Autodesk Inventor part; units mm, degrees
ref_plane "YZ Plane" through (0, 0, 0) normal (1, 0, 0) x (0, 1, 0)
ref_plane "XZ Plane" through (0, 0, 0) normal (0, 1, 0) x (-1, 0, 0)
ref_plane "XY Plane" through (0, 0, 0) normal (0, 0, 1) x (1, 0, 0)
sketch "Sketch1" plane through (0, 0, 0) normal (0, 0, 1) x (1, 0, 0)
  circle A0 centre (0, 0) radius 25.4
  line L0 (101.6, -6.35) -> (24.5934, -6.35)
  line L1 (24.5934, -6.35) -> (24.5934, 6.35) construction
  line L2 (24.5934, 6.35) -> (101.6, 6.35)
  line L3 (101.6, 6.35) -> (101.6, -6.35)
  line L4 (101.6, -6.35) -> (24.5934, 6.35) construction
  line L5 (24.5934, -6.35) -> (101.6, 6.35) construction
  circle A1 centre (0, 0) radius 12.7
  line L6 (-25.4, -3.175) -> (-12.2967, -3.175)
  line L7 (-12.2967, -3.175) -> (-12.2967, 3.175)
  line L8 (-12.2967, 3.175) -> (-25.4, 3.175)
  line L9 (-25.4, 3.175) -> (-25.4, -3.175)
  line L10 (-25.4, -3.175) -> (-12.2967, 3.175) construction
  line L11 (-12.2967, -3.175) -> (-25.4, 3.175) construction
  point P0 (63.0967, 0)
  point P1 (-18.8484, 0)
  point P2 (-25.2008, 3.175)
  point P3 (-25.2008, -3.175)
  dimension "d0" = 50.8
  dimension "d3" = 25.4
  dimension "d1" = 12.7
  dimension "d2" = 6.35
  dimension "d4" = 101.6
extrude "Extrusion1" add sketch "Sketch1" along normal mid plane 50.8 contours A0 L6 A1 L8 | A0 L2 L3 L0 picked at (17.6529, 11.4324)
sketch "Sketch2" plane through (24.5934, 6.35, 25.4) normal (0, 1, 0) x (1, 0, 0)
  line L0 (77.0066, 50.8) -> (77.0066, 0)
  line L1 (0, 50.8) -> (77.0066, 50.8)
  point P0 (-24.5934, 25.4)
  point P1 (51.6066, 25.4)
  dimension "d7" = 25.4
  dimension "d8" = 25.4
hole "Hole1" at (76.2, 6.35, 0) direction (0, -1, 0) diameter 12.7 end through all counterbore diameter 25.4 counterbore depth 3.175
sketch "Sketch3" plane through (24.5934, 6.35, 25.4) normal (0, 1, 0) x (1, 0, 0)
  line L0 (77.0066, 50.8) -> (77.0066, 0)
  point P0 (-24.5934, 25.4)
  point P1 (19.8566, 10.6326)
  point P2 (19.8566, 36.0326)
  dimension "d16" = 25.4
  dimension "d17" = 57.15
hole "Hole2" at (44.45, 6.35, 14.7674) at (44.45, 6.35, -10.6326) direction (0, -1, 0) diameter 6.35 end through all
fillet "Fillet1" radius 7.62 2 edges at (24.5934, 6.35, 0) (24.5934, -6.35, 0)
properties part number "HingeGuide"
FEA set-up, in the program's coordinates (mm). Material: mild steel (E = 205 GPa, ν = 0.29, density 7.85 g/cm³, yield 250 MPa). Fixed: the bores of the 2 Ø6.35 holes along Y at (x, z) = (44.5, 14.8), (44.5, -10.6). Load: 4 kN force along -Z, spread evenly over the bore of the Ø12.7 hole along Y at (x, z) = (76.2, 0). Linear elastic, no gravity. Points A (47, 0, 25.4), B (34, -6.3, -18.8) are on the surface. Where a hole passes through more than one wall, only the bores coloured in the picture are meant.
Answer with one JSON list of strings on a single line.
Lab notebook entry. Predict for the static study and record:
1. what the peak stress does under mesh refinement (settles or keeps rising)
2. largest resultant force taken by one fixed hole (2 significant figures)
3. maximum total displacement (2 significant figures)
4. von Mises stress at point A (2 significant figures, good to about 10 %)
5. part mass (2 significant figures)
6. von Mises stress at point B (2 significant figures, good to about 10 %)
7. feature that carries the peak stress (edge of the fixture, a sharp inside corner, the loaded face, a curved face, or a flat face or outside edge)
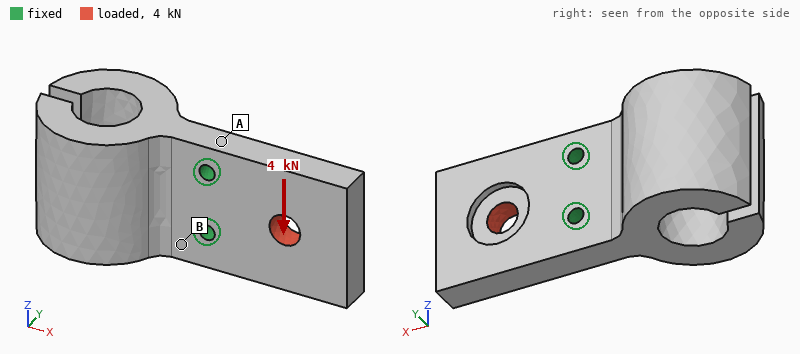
["keeps rising", "4.7 kN", "10 µm", "17 MPa", "940 g", "5.4 MPa", "edge of the fixture"]
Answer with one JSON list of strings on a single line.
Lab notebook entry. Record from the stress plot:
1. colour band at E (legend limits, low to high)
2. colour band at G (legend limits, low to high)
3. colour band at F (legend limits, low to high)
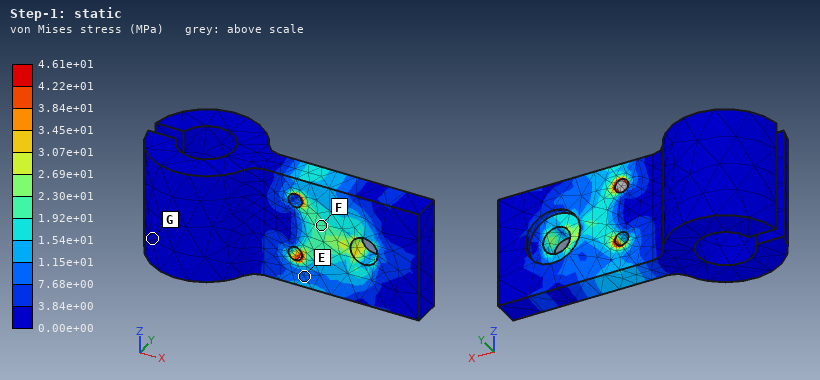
["7.68e+00 to 1.15e+01 MPa", "0.00e+00 to 3.84e+00 MPa", "1.92e+01 to 2.30e+01 MPa"]
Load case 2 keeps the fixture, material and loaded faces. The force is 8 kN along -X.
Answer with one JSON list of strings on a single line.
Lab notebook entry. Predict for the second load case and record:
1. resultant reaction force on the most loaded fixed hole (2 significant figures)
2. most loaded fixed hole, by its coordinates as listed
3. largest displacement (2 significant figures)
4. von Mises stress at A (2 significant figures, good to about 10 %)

["4.6 kN", "(44.5, -10.6)", "9.9 µm", "8.2 MPa"]
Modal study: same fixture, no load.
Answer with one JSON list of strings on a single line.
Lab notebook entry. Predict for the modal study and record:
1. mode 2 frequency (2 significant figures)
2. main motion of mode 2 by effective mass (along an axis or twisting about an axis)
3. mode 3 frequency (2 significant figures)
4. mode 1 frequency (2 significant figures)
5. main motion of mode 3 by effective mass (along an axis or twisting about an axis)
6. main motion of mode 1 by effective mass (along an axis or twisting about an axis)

["3000 Hz", "along Y", "3900 Hz", "1400 Hz", "along Z", "along Y"]
